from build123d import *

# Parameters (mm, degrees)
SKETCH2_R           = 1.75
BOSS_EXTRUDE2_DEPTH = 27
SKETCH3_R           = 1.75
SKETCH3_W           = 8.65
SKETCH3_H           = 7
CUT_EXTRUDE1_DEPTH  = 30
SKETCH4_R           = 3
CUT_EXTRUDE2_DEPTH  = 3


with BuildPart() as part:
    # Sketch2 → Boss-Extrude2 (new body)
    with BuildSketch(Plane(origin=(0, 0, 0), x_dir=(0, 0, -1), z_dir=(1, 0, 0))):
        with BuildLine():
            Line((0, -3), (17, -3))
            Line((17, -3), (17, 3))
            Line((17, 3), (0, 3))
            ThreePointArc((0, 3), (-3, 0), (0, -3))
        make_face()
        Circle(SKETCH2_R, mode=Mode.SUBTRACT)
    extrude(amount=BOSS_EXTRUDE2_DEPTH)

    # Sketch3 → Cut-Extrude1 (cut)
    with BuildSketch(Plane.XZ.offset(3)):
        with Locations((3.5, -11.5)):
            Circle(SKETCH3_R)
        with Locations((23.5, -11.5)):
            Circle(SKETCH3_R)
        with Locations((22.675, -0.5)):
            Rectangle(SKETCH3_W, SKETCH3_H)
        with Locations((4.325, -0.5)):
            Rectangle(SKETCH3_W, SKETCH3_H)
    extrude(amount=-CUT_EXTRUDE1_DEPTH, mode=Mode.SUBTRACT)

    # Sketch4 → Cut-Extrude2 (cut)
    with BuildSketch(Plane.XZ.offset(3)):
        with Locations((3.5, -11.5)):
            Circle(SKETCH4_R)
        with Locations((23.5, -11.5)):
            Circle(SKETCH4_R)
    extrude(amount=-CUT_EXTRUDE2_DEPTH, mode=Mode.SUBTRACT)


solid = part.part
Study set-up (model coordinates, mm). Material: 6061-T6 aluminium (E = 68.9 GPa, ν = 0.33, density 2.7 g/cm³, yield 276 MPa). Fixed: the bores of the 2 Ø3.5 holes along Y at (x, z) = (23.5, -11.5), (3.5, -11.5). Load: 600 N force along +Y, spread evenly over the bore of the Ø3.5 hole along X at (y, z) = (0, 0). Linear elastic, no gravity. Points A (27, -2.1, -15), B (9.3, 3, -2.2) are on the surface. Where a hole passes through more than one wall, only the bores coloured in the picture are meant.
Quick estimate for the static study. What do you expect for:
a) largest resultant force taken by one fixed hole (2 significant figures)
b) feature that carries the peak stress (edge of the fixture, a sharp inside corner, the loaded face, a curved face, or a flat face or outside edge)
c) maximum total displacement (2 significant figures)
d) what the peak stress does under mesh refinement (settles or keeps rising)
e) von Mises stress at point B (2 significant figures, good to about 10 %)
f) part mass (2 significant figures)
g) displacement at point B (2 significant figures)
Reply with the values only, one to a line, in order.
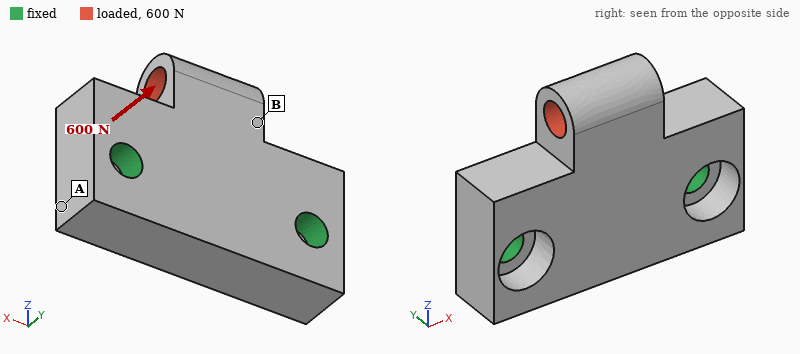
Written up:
360 N
edge of the fixture
67 µm
keeps rising
54 MPa
5.8 g
37 µm
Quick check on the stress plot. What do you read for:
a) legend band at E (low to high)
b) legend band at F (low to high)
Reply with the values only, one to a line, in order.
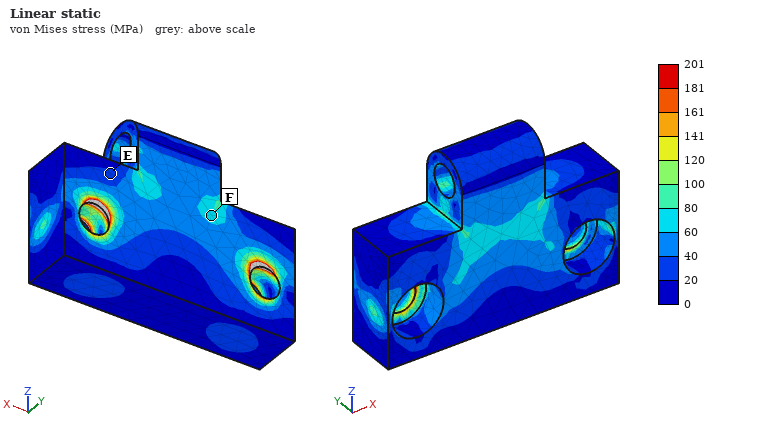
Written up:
20 to 40 MPa
60 to 80 MPa
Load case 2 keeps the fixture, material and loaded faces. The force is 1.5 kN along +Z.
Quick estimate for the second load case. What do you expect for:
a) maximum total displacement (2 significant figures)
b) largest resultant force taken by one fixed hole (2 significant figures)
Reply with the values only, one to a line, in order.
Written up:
17 µm
780 N
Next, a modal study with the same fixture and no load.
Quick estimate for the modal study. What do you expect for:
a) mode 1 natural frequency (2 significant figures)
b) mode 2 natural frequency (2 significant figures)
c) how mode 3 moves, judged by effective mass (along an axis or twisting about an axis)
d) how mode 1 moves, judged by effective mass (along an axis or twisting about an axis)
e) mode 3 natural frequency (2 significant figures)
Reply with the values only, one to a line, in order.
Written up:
18 kHz
40 kHz
along Z
along Y
48 kHz
